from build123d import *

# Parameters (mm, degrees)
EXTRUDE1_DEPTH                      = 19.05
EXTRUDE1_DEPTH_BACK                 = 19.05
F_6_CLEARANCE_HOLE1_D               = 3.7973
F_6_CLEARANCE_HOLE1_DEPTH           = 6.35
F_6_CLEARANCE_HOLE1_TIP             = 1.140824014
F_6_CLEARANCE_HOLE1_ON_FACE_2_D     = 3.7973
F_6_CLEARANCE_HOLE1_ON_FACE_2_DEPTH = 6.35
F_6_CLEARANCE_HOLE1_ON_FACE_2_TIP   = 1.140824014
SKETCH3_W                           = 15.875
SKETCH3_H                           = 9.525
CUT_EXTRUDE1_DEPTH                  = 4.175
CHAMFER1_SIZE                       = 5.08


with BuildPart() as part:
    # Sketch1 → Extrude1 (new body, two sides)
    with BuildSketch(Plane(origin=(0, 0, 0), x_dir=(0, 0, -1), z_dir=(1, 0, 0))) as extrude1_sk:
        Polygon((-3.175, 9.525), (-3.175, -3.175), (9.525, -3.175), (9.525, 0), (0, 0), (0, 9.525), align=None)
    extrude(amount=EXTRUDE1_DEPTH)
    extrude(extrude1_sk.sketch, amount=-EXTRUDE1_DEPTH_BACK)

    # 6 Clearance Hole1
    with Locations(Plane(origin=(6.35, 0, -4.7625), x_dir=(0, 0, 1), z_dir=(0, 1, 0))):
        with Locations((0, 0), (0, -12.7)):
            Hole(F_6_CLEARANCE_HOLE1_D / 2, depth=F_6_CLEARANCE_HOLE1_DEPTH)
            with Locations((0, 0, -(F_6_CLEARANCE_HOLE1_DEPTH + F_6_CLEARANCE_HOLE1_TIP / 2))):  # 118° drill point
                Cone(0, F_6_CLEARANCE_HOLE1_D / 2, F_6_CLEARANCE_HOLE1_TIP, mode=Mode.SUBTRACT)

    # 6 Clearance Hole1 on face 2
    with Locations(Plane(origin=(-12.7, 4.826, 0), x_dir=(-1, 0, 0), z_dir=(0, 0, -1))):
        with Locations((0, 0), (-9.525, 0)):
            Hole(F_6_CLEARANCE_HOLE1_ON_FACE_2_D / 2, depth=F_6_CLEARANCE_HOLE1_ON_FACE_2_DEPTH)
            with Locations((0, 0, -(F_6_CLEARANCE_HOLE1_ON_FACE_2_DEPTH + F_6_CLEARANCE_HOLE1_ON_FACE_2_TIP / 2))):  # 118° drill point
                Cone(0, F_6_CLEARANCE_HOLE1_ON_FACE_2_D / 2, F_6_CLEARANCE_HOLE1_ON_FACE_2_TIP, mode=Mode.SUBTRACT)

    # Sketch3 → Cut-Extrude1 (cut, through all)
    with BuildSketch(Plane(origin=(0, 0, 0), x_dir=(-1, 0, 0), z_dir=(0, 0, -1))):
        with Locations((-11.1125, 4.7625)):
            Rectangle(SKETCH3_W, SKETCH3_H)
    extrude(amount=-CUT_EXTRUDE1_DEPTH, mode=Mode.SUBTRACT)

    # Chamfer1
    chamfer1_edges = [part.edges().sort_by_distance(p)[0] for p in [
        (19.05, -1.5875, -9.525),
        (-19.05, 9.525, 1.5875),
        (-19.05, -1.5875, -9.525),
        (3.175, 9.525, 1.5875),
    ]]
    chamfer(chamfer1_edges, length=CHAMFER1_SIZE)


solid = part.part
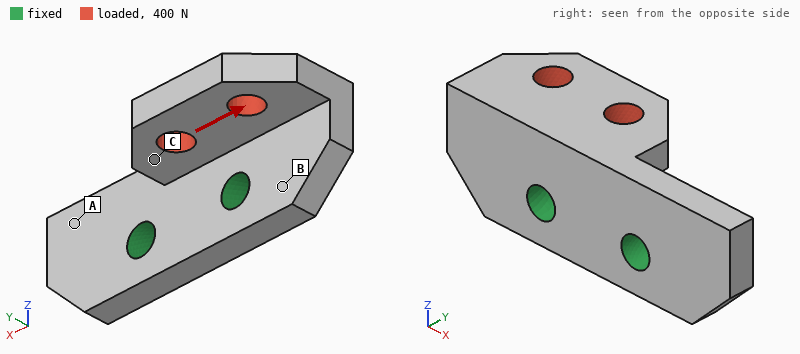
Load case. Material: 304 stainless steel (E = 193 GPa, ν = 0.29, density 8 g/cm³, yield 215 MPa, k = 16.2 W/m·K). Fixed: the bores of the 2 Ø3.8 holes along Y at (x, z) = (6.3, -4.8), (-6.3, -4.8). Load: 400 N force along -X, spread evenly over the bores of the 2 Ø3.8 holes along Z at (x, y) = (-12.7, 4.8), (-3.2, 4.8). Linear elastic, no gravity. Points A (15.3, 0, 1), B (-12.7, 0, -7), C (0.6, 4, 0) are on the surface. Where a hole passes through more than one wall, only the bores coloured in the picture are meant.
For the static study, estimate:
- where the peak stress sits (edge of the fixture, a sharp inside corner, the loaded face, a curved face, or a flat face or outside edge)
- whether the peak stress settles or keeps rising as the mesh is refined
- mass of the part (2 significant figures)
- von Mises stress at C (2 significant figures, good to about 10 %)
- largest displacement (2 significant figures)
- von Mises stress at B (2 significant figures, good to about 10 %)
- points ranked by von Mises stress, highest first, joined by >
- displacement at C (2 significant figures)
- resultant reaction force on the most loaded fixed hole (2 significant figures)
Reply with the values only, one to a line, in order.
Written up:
edge of the fixture
keeps rising
15 g
24 MPa
7.6 µm
13 MPa
C > B > A
3.0 µm
310 N
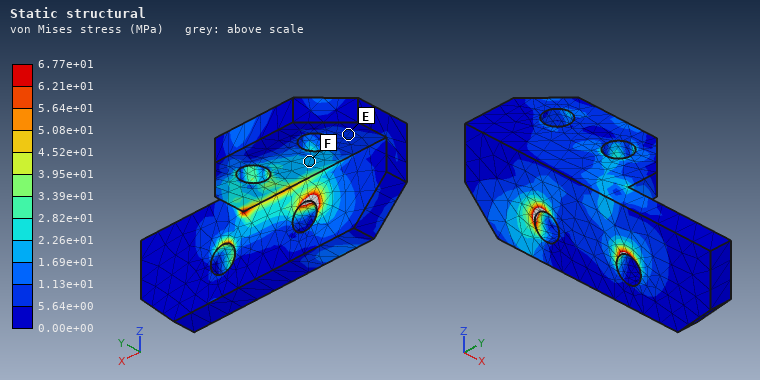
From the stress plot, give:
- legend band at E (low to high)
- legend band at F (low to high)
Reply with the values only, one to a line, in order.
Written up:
5.64e+00 to 1.13e+01 MPa
1.69e+01 to 2.26e+01 MPa
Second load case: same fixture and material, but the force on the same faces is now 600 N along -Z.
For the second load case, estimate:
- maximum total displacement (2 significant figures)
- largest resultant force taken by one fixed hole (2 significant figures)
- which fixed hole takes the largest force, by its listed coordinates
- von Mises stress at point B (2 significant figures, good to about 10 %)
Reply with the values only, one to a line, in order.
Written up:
35 µm
600 N
(-6.3, -4.8)
42 MPa
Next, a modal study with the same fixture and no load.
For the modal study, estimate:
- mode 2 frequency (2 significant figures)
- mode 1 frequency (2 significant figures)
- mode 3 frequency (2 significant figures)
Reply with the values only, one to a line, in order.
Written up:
18 kHz
12 kHz
18 kHz
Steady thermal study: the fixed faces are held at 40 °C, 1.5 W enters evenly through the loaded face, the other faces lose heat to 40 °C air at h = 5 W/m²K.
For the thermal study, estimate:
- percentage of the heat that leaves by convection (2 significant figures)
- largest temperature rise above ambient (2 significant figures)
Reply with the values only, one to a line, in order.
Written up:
3.3 %
20 K
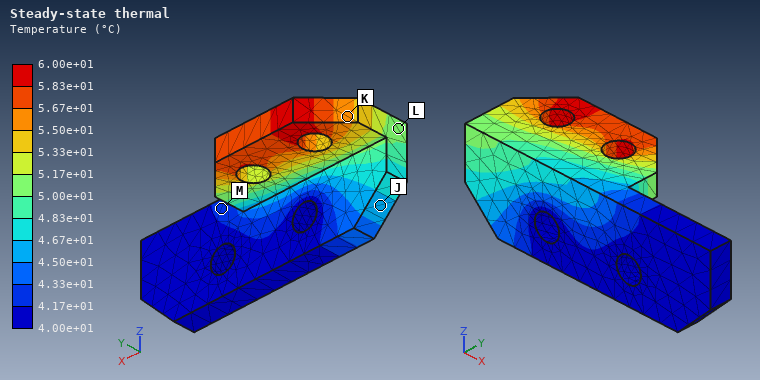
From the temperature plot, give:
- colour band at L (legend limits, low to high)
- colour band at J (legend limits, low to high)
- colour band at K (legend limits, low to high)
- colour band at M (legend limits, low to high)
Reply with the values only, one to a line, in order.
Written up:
5.00e+01 to 5.17e+01 °C
4.50e+01 to 4.67e+01 °C
5.50e+01 to 5.67e+01 °C
4.17e+01 to 4.33e+01 °C
